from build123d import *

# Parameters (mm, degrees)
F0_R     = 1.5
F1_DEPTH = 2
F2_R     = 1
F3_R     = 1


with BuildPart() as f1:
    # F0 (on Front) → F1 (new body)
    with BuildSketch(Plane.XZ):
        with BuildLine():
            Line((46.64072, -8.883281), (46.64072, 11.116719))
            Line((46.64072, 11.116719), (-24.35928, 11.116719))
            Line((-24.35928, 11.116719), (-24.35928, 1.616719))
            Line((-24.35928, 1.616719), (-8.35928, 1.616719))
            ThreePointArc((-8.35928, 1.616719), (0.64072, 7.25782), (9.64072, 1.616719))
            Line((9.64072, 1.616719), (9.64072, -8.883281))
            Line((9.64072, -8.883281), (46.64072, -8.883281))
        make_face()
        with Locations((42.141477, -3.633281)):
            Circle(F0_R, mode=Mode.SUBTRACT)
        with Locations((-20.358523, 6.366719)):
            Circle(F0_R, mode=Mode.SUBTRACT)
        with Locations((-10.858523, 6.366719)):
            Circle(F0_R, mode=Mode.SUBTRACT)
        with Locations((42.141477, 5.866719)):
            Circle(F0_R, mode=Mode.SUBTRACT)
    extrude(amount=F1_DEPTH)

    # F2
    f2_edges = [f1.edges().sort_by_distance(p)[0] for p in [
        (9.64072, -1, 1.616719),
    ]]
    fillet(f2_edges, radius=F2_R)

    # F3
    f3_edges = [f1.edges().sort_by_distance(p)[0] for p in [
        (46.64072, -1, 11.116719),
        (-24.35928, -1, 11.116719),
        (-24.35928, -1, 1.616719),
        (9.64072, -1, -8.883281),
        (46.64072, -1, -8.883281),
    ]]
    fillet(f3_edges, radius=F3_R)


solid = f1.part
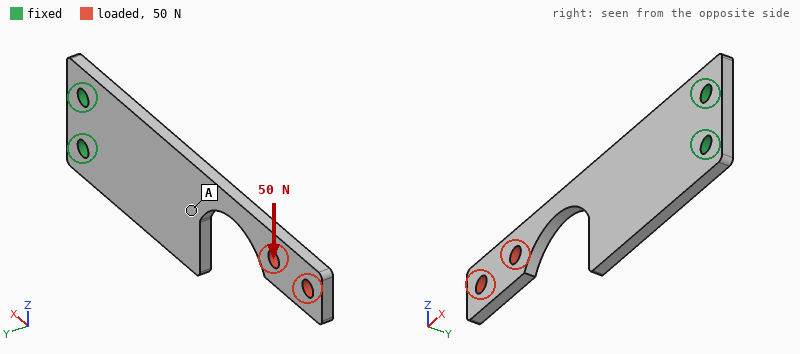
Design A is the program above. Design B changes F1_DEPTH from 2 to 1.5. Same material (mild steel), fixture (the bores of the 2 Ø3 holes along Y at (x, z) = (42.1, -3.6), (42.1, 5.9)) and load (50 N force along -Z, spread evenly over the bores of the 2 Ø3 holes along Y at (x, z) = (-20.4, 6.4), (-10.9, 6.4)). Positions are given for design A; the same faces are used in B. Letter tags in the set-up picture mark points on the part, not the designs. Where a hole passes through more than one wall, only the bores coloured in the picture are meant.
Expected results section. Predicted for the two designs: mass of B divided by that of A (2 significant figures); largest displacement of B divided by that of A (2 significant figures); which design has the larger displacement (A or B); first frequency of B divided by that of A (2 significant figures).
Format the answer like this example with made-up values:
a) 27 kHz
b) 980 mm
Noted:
a) 0.75
b) 1.3
c) B
d) 0.75
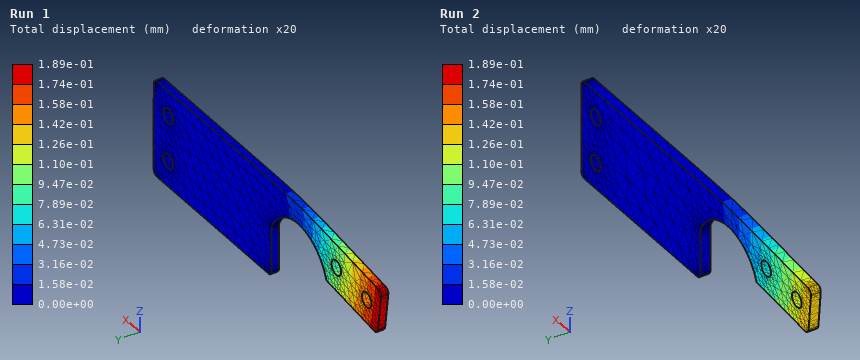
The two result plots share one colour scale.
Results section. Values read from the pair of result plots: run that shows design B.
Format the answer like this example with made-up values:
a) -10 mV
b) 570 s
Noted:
a) Run 1
